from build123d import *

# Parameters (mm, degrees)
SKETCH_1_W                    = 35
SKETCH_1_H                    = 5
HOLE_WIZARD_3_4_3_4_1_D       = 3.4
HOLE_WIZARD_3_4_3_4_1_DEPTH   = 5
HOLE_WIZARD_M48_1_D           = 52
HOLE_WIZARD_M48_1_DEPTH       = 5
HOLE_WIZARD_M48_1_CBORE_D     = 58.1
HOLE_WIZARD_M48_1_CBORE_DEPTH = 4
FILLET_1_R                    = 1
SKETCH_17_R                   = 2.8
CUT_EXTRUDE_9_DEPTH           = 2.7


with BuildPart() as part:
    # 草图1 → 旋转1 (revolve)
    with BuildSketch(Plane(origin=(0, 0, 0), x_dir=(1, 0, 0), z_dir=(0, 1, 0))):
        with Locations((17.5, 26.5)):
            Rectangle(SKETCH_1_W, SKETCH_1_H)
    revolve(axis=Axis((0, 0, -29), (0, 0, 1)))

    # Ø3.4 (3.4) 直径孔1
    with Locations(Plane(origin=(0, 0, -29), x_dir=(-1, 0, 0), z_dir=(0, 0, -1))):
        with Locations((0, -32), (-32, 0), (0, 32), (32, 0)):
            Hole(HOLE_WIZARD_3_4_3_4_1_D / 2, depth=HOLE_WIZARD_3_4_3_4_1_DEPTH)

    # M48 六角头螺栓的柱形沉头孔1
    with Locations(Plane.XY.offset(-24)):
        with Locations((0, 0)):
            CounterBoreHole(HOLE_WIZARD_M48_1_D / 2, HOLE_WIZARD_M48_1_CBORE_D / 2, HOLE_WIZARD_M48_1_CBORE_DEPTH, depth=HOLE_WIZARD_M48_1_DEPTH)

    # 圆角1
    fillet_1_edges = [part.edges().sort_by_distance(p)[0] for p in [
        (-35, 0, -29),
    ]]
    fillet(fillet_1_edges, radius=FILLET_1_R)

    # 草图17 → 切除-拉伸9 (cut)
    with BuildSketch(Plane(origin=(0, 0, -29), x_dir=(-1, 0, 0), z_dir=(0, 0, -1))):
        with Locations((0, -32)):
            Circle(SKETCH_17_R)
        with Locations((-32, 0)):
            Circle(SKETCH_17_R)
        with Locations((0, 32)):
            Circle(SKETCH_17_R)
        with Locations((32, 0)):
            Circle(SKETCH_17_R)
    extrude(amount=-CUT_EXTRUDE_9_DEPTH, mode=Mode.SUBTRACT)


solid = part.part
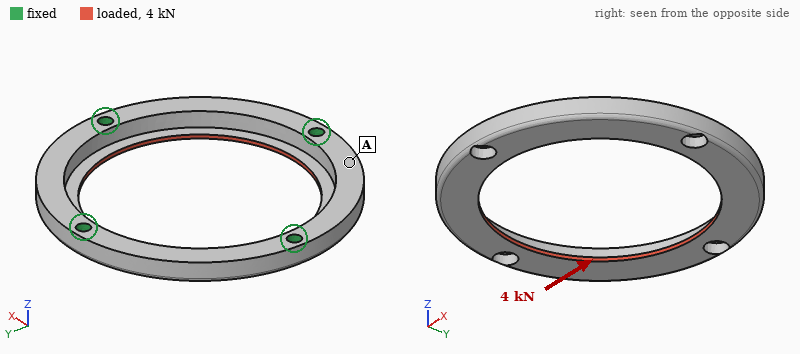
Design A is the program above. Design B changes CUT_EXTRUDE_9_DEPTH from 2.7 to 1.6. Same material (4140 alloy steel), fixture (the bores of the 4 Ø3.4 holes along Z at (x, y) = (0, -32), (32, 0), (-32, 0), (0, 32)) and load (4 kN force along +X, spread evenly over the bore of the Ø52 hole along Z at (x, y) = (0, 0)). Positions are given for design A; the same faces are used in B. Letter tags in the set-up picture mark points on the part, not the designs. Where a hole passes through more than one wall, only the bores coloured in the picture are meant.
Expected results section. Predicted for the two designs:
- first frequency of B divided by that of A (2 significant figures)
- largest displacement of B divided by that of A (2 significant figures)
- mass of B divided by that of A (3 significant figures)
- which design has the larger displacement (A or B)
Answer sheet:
1.2
0.64
1.01
A
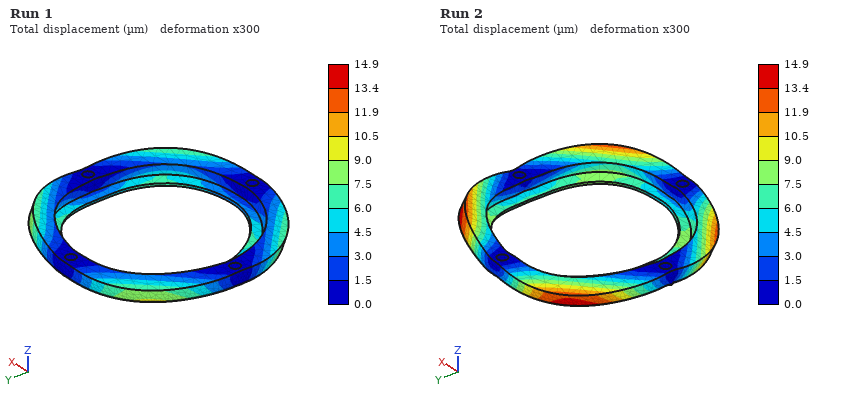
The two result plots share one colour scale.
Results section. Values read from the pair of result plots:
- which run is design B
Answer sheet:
Run 1
